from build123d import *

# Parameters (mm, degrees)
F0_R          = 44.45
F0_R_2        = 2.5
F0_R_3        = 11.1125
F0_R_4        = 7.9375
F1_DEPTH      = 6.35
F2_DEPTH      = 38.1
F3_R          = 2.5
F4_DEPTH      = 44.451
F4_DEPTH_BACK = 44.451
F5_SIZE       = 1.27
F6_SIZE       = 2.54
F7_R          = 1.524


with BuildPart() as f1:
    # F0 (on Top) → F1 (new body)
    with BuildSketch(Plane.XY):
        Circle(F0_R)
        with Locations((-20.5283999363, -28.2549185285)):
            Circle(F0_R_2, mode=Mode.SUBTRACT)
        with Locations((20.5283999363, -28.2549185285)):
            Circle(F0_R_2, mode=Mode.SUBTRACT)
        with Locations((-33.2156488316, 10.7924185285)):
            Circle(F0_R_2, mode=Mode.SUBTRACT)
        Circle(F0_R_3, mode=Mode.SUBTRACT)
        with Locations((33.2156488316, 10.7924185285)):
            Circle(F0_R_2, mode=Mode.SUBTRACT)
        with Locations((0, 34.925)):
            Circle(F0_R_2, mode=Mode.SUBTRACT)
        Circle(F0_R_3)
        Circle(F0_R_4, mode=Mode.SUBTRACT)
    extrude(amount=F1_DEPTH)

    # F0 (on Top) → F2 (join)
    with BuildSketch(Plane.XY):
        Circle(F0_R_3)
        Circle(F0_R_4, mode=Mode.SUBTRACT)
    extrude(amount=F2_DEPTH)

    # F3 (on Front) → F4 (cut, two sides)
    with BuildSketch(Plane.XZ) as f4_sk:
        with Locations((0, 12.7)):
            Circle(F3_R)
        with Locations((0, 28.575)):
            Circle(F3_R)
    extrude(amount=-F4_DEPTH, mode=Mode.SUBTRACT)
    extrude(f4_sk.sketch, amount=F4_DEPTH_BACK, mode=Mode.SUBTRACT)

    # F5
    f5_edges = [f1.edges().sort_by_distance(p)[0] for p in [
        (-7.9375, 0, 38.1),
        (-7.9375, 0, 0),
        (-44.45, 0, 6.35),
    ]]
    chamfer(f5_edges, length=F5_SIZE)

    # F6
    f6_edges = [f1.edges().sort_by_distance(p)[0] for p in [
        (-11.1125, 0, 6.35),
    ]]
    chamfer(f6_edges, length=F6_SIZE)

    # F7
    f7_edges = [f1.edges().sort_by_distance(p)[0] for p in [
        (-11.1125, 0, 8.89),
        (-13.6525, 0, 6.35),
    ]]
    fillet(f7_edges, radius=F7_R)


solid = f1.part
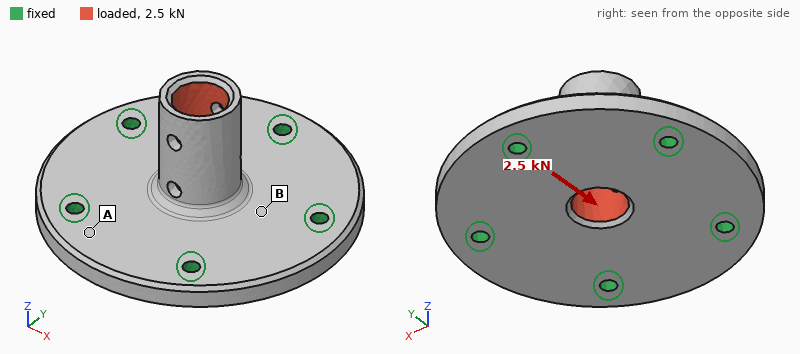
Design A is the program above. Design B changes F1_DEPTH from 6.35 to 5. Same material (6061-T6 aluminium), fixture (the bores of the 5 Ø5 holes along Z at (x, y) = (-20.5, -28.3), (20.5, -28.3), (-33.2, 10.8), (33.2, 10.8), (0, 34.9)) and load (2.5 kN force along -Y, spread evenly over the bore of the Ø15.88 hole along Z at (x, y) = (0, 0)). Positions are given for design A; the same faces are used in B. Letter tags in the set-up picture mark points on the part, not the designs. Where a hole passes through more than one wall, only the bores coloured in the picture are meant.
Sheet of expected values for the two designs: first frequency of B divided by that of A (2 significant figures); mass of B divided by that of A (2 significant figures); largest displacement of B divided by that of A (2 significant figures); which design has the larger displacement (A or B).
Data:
0.81
0.82
1.6
B
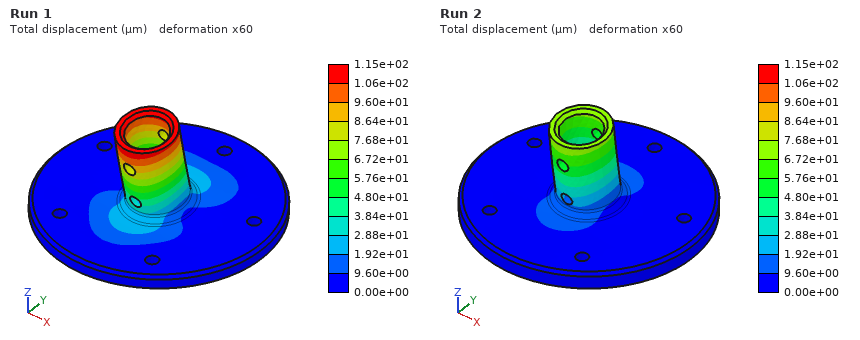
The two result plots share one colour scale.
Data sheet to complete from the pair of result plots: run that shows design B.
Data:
Run 1
